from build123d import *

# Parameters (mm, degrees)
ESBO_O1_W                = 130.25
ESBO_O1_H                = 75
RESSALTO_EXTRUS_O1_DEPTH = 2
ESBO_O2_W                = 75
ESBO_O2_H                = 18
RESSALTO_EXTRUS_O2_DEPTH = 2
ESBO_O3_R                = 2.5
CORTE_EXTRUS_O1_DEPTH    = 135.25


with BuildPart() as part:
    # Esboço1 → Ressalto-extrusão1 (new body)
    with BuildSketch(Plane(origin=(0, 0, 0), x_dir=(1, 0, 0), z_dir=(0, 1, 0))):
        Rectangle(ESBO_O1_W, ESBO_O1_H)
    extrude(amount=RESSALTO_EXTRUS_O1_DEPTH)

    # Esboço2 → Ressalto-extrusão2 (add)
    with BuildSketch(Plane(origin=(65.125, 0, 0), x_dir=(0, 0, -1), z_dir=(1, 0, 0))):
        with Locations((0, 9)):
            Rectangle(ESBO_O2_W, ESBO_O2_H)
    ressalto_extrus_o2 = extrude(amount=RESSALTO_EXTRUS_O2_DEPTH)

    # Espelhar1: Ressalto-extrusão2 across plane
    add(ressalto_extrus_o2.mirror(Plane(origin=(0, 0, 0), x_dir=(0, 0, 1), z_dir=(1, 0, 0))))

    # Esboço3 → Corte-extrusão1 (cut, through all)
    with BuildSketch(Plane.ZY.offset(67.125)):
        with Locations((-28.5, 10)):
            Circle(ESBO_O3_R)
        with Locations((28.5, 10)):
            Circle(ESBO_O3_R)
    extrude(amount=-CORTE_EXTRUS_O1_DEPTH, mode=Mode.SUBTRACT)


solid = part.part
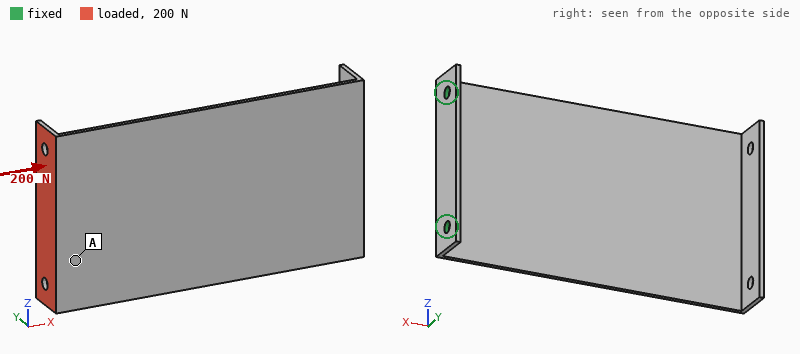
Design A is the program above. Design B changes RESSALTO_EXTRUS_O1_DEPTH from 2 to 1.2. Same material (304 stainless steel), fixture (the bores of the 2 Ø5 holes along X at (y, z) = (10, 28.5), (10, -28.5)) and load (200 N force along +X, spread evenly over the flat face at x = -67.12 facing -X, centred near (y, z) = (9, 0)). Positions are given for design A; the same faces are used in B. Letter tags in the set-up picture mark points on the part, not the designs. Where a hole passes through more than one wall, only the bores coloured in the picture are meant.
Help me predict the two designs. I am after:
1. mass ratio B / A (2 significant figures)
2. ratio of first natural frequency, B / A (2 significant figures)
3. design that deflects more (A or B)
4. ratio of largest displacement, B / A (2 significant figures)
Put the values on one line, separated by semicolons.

0.68; 0.60; B; 4.6
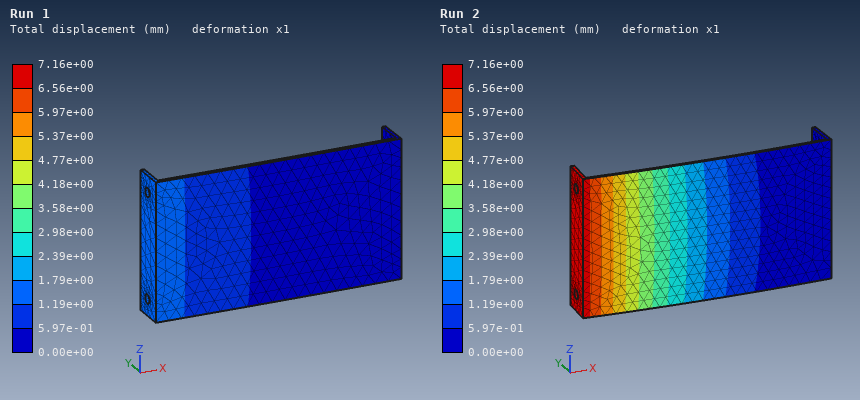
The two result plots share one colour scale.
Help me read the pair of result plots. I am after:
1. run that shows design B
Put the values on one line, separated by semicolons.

Run 2
